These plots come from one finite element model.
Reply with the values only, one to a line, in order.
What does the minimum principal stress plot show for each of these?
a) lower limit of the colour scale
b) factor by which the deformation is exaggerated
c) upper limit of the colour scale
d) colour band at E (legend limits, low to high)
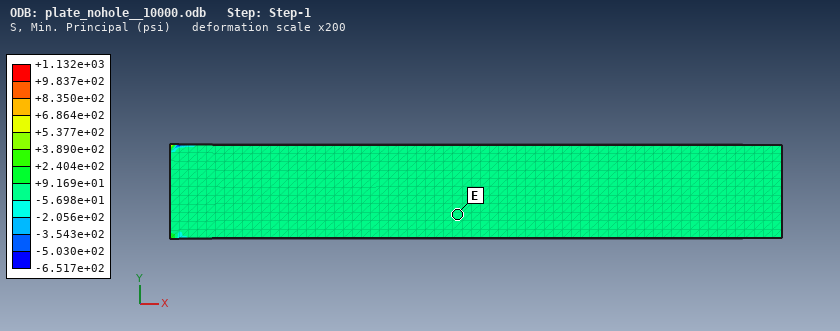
-6.517e+02 psi
200
+1.132e+03 psi
-5.698e+01 to +9.169e+01 psi
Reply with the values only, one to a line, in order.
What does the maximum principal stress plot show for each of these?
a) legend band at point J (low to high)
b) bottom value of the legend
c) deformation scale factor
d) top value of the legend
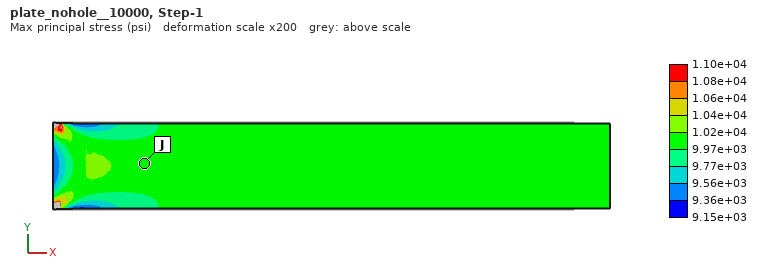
9.97e+03 to 1.02e+04 psi
9.15e+03 psi
200
1.10e+04 psi
